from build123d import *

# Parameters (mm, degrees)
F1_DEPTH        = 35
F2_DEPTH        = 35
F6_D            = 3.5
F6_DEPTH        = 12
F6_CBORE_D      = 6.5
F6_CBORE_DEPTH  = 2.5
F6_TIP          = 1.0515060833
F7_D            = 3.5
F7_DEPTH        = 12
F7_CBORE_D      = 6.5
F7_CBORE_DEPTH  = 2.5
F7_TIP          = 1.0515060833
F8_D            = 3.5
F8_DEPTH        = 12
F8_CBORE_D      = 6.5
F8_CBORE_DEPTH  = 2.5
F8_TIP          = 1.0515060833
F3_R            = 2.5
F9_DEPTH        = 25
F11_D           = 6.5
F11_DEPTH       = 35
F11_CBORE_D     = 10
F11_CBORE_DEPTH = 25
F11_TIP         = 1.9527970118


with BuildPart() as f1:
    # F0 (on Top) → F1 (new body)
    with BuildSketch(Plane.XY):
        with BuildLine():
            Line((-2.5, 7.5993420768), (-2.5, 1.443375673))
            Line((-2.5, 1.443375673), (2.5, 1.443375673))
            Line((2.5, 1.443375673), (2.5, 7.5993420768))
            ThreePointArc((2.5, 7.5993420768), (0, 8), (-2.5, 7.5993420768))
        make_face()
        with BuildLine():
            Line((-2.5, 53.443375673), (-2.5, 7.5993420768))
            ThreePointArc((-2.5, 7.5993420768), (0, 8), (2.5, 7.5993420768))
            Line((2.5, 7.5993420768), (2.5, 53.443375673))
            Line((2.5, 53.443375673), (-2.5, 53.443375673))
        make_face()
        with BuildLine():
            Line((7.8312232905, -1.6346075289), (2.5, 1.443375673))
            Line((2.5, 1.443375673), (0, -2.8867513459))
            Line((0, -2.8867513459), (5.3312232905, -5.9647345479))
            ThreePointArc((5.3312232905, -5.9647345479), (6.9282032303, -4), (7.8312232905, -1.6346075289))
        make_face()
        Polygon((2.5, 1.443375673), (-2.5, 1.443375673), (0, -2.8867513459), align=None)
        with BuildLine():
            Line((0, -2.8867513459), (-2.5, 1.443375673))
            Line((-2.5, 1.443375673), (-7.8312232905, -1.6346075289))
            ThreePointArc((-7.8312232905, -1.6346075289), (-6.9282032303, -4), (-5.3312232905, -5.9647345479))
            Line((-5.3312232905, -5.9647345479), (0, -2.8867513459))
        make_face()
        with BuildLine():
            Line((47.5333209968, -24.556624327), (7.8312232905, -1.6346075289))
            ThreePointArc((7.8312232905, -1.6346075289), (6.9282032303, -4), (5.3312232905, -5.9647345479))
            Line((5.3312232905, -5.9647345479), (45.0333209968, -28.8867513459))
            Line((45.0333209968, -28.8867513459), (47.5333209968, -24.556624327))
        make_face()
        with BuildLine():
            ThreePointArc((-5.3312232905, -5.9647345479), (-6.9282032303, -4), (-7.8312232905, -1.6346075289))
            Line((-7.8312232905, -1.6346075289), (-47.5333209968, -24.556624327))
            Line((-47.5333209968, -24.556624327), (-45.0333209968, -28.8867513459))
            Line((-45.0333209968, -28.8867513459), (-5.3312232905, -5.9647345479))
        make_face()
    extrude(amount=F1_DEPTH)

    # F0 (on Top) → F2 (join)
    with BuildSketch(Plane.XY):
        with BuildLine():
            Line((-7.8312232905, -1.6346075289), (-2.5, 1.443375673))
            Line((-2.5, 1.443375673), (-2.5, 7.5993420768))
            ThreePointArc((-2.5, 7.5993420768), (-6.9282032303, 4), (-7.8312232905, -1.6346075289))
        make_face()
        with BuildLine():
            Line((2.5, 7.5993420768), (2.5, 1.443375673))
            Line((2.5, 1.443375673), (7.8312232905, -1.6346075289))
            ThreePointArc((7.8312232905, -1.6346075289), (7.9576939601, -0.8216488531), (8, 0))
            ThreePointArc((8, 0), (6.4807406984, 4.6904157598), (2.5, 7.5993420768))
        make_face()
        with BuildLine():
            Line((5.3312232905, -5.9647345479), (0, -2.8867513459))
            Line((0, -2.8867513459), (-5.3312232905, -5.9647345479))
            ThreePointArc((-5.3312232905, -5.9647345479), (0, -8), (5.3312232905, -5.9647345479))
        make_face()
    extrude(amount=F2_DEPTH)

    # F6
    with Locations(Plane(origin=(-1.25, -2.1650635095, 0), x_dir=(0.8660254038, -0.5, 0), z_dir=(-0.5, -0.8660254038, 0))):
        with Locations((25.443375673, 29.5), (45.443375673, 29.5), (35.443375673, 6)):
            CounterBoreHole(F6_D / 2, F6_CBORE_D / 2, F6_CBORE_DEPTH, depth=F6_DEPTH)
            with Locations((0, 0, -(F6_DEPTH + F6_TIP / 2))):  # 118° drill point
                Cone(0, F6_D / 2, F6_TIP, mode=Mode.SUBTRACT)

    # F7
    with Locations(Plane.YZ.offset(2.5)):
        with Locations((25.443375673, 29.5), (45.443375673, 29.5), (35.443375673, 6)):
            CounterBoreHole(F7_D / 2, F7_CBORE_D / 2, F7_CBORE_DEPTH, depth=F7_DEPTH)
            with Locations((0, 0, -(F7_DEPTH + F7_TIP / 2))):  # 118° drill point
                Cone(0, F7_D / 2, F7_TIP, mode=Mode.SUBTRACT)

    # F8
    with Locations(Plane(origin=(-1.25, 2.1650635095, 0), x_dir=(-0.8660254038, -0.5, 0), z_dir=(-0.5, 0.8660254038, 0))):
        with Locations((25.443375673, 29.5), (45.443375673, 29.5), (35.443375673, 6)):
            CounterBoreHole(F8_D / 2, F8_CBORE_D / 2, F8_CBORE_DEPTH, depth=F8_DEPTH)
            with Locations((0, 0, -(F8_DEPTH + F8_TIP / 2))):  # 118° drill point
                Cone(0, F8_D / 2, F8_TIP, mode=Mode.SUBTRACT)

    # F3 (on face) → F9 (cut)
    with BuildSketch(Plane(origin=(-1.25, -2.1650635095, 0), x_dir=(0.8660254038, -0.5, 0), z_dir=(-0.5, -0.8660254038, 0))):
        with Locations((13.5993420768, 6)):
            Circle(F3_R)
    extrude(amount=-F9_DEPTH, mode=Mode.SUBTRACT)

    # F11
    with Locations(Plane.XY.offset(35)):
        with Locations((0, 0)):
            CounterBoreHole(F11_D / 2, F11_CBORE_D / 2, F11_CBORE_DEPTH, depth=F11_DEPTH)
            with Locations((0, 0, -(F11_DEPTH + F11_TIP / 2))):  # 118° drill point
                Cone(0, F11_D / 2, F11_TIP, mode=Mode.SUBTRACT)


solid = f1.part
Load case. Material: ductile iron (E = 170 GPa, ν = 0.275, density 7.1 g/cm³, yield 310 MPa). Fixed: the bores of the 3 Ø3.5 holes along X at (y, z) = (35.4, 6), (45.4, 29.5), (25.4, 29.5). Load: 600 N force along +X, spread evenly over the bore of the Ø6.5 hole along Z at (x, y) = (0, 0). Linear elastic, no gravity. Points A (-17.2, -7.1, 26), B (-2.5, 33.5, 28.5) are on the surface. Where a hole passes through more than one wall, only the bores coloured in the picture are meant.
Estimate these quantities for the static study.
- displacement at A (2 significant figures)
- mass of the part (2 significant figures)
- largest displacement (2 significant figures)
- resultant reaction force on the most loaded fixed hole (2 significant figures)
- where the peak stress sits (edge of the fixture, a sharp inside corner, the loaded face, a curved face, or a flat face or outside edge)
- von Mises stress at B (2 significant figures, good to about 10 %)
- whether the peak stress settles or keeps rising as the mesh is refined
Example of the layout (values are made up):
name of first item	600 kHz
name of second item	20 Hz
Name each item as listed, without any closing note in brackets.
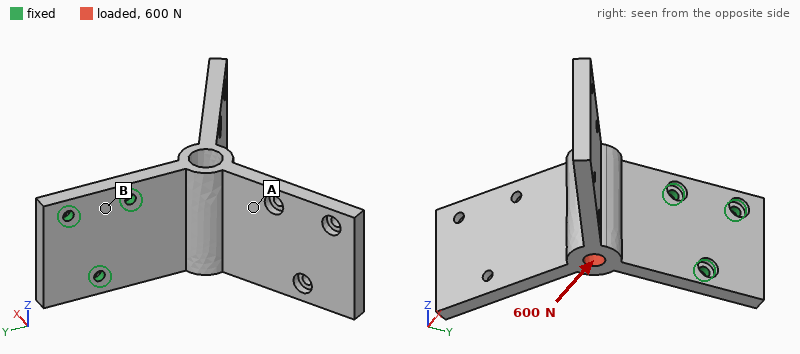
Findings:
displacement at A	0.18 mm
mass of the part	200 g
largest displacement	0.44 mm
resultant reaction force on the most loaded fixed hole	1.1 kN
where the peak stress sits	edge of the fixture
von Mises stress at B	31 MPa
whether the peak stress settles or keeps rising as the mesh is refined	keeps rising
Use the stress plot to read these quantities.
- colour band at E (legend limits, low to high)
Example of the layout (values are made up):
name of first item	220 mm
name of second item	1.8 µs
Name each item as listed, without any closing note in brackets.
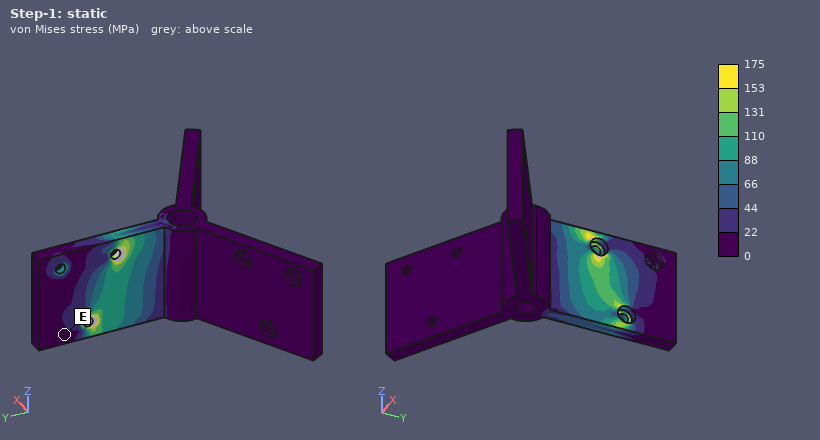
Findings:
colour band at E	0 to 22 MPa
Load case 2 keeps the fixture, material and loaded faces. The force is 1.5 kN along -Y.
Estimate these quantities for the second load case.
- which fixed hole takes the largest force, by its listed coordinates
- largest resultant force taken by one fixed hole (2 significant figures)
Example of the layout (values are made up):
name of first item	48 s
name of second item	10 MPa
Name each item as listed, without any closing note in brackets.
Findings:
which fixed hole takes the largest force, by its listed coordinates	(35.4, 6)
largest resultant force taken by one fixed hole	1.3 kN
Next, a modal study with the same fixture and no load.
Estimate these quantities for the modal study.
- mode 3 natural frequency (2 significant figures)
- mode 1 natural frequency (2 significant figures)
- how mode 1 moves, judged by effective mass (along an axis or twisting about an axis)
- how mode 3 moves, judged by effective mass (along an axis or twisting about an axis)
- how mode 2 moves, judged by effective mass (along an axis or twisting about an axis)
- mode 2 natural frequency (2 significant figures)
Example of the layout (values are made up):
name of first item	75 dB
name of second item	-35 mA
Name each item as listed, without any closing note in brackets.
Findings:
mode 3 natural frequency	1600 Hz
mode 1 natural frequency	460 Hz
how mode 1 moves, judged by effective mass	along X
how mode 3 moves, judged by effective mass	along Y
how mode 2 moves, judged by effective mass	twisting about Y
mode 2 natural frequency	1200 Hz
